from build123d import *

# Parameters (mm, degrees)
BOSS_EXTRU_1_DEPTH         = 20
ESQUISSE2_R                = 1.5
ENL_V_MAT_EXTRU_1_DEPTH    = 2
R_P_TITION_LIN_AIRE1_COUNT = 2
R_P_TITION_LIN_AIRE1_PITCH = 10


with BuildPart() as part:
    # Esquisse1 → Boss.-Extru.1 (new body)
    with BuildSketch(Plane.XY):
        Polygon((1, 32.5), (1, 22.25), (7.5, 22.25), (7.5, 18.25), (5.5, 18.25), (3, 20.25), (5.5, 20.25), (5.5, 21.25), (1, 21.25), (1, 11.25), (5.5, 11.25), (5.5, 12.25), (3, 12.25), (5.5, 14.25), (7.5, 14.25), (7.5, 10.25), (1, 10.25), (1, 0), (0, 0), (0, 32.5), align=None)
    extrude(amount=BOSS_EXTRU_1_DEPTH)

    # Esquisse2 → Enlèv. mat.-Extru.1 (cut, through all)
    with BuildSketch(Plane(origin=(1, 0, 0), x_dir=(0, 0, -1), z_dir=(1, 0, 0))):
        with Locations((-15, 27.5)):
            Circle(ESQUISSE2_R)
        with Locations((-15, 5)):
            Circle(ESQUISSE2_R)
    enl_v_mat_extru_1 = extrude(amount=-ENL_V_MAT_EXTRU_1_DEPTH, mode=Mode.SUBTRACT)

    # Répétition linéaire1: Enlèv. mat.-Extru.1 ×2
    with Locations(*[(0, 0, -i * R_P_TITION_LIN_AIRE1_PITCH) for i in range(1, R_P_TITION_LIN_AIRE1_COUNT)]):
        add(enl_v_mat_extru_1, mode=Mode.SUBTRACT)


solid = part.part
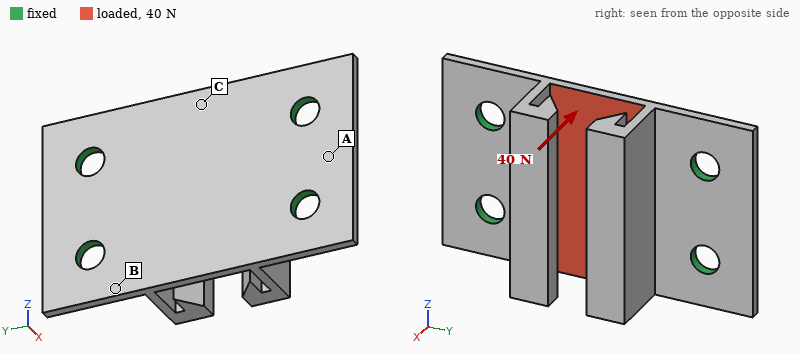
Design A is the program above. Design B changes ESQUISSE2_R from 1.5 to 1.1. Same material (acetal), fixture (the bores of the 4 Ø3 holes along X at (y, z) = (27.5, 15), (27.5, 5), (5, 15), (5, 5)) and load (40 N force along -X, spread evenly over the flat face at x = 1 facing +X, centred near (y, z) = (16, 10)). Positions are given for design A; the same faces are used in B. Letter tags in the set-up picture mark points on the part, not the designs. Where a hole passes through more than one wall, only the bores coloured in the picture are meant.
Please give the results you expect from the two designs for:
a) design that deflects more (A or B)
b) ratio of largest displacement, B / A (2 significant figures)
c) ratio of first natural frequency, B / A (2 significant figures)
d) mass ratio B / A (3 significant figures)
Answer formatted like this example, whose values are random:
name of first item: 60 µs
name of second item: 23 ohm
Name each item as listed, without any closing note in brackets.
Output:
design that deflects more: B
ratio of largest displacement, B / A: 1.1
ratio of first natural frequency, B / A: 0.96
mass ratio B / A: 1.01
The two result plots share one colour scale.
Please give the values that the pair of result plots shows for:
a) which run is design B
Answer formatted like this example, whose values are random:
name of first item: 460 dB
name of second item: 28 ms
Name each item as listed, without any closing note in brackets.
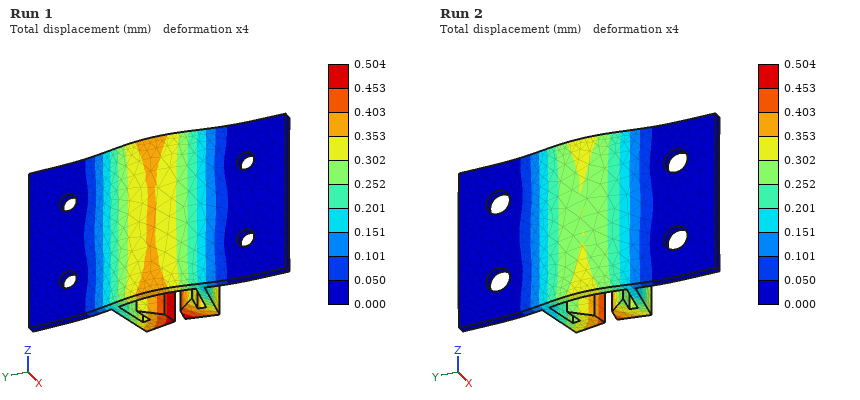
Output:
which run is design B: Run 1
